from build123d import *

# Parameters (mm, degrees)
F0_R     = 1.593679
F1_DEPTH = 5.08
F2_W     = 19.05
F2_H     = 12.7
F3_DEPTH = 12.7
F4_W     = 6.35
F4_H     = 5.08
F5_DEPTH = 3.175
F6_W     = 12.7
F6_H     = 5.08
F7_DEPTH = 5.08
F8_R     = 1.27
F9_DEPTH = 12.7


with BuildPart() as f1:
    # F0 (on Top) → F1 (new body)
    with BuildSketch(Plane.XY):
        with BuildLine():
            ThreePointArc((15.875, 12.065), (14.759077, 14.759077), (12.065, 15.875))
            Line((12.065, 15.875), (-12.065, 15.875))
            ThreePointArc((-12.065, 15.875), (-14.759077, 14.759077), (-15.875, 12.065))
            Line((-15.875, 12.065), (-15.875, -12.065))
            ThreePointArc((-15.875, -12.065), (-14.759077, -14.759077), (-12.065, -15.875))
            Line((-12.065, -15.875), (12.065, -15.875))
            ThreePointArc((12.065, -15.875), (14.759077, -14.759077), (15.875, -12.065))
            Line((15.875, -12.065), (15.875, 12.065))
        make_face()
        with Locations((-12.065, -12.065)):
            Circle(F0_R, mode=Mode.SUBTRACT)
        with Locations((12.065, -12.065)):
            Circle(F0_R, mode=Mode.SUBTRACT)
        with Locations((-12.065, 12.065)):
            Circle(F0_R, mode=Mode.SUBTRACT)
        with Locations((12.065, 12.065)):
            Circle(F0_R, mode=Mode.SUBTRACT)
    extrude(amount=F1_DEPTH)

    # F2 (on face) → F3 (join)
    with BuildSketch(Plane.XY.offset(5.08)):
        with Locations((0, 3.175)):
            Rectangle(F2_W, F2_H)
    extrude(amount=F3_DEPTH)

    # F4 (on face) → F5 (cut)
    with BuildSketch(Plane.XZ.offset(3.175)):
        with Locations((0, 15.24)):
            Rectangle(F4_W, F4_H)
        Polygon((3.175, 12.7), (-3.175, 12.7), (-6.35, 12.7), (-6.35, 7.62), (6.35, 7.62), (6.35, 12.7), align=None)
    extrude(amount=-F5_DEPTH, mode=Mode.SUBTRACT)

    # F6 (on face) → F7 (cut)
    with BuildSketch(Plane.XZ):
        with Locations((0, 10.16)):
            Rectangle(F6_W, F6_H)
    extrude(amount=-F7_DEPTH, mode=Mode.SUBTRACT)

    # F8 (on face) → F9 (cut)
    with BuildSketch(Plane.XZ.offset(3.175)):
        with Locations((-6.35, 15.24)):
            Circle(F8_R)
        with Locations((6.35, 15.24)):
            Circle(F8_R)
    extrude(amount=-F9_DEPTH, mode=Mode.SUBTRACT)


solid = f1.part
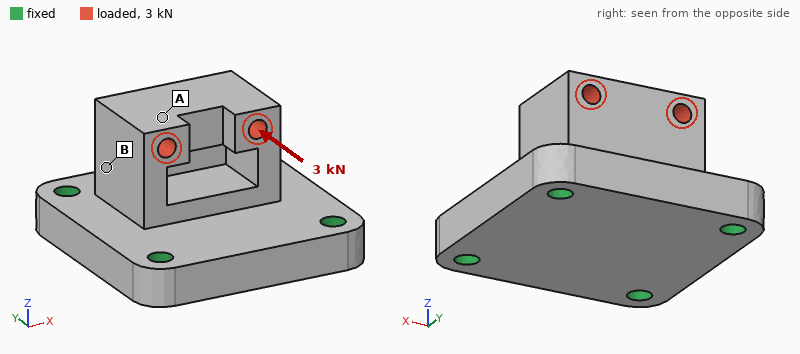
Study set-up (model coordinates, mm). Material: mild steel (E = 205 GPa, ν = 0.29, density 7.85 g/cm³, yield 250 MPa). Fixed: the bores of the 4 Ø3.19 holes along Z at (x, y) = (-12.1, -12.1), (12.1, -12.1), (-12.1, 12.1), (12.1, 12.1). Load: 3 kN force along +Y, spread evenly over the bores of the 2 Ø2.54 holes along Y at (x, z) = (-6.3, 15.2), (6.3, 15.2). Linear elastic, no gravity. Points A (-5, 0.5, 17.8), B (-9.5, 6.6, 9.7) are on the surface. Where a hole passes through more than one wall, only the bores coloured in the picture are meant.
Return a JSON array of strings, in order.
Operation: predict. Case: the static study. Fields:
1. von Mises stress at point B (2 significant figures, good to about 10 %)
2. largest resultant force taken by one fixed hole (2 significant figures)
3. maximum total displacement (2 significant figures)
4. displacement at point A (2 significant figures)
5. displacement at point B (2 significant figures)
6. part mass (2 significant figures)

["55 MPa", "1.3 kN", "21 µm", "19 µm", "6.8 µm", "57 g"]
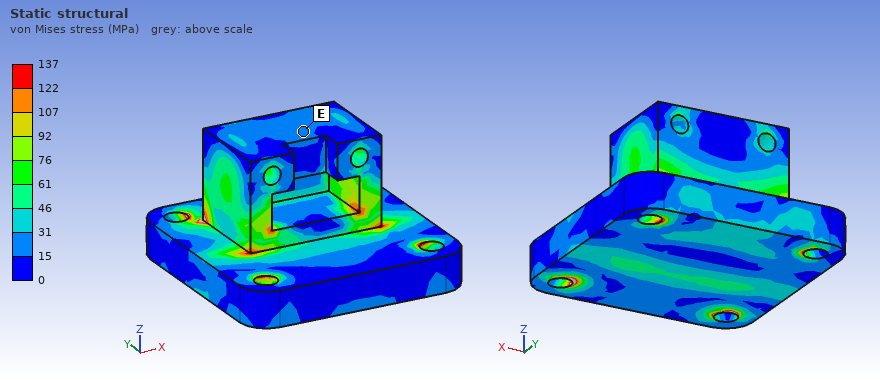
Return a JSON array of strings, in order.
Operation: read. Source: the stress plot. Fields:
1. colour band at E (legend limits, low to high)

["15 to 31 MPa"]
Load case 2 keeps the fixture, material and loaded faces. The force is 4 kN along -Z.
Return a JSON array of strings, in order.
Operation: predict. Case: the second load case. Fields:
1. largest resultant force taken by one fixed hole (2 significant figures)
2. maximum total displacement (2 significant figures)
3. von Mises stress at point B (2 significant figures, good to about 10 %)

["1.3 kN", "11 µm", "26 MPa"]
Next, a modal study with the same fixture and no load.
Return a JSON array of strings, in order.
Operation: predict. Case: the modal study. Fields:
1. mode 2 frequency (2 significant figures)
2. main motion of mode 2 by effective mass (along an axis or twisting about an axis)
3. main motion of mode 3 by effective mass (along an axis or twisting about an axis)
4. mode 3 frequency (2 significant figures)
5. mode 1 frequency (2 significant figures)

["24 kHz", "along X", "along Z", "26 kHz", "20 kHz"]
